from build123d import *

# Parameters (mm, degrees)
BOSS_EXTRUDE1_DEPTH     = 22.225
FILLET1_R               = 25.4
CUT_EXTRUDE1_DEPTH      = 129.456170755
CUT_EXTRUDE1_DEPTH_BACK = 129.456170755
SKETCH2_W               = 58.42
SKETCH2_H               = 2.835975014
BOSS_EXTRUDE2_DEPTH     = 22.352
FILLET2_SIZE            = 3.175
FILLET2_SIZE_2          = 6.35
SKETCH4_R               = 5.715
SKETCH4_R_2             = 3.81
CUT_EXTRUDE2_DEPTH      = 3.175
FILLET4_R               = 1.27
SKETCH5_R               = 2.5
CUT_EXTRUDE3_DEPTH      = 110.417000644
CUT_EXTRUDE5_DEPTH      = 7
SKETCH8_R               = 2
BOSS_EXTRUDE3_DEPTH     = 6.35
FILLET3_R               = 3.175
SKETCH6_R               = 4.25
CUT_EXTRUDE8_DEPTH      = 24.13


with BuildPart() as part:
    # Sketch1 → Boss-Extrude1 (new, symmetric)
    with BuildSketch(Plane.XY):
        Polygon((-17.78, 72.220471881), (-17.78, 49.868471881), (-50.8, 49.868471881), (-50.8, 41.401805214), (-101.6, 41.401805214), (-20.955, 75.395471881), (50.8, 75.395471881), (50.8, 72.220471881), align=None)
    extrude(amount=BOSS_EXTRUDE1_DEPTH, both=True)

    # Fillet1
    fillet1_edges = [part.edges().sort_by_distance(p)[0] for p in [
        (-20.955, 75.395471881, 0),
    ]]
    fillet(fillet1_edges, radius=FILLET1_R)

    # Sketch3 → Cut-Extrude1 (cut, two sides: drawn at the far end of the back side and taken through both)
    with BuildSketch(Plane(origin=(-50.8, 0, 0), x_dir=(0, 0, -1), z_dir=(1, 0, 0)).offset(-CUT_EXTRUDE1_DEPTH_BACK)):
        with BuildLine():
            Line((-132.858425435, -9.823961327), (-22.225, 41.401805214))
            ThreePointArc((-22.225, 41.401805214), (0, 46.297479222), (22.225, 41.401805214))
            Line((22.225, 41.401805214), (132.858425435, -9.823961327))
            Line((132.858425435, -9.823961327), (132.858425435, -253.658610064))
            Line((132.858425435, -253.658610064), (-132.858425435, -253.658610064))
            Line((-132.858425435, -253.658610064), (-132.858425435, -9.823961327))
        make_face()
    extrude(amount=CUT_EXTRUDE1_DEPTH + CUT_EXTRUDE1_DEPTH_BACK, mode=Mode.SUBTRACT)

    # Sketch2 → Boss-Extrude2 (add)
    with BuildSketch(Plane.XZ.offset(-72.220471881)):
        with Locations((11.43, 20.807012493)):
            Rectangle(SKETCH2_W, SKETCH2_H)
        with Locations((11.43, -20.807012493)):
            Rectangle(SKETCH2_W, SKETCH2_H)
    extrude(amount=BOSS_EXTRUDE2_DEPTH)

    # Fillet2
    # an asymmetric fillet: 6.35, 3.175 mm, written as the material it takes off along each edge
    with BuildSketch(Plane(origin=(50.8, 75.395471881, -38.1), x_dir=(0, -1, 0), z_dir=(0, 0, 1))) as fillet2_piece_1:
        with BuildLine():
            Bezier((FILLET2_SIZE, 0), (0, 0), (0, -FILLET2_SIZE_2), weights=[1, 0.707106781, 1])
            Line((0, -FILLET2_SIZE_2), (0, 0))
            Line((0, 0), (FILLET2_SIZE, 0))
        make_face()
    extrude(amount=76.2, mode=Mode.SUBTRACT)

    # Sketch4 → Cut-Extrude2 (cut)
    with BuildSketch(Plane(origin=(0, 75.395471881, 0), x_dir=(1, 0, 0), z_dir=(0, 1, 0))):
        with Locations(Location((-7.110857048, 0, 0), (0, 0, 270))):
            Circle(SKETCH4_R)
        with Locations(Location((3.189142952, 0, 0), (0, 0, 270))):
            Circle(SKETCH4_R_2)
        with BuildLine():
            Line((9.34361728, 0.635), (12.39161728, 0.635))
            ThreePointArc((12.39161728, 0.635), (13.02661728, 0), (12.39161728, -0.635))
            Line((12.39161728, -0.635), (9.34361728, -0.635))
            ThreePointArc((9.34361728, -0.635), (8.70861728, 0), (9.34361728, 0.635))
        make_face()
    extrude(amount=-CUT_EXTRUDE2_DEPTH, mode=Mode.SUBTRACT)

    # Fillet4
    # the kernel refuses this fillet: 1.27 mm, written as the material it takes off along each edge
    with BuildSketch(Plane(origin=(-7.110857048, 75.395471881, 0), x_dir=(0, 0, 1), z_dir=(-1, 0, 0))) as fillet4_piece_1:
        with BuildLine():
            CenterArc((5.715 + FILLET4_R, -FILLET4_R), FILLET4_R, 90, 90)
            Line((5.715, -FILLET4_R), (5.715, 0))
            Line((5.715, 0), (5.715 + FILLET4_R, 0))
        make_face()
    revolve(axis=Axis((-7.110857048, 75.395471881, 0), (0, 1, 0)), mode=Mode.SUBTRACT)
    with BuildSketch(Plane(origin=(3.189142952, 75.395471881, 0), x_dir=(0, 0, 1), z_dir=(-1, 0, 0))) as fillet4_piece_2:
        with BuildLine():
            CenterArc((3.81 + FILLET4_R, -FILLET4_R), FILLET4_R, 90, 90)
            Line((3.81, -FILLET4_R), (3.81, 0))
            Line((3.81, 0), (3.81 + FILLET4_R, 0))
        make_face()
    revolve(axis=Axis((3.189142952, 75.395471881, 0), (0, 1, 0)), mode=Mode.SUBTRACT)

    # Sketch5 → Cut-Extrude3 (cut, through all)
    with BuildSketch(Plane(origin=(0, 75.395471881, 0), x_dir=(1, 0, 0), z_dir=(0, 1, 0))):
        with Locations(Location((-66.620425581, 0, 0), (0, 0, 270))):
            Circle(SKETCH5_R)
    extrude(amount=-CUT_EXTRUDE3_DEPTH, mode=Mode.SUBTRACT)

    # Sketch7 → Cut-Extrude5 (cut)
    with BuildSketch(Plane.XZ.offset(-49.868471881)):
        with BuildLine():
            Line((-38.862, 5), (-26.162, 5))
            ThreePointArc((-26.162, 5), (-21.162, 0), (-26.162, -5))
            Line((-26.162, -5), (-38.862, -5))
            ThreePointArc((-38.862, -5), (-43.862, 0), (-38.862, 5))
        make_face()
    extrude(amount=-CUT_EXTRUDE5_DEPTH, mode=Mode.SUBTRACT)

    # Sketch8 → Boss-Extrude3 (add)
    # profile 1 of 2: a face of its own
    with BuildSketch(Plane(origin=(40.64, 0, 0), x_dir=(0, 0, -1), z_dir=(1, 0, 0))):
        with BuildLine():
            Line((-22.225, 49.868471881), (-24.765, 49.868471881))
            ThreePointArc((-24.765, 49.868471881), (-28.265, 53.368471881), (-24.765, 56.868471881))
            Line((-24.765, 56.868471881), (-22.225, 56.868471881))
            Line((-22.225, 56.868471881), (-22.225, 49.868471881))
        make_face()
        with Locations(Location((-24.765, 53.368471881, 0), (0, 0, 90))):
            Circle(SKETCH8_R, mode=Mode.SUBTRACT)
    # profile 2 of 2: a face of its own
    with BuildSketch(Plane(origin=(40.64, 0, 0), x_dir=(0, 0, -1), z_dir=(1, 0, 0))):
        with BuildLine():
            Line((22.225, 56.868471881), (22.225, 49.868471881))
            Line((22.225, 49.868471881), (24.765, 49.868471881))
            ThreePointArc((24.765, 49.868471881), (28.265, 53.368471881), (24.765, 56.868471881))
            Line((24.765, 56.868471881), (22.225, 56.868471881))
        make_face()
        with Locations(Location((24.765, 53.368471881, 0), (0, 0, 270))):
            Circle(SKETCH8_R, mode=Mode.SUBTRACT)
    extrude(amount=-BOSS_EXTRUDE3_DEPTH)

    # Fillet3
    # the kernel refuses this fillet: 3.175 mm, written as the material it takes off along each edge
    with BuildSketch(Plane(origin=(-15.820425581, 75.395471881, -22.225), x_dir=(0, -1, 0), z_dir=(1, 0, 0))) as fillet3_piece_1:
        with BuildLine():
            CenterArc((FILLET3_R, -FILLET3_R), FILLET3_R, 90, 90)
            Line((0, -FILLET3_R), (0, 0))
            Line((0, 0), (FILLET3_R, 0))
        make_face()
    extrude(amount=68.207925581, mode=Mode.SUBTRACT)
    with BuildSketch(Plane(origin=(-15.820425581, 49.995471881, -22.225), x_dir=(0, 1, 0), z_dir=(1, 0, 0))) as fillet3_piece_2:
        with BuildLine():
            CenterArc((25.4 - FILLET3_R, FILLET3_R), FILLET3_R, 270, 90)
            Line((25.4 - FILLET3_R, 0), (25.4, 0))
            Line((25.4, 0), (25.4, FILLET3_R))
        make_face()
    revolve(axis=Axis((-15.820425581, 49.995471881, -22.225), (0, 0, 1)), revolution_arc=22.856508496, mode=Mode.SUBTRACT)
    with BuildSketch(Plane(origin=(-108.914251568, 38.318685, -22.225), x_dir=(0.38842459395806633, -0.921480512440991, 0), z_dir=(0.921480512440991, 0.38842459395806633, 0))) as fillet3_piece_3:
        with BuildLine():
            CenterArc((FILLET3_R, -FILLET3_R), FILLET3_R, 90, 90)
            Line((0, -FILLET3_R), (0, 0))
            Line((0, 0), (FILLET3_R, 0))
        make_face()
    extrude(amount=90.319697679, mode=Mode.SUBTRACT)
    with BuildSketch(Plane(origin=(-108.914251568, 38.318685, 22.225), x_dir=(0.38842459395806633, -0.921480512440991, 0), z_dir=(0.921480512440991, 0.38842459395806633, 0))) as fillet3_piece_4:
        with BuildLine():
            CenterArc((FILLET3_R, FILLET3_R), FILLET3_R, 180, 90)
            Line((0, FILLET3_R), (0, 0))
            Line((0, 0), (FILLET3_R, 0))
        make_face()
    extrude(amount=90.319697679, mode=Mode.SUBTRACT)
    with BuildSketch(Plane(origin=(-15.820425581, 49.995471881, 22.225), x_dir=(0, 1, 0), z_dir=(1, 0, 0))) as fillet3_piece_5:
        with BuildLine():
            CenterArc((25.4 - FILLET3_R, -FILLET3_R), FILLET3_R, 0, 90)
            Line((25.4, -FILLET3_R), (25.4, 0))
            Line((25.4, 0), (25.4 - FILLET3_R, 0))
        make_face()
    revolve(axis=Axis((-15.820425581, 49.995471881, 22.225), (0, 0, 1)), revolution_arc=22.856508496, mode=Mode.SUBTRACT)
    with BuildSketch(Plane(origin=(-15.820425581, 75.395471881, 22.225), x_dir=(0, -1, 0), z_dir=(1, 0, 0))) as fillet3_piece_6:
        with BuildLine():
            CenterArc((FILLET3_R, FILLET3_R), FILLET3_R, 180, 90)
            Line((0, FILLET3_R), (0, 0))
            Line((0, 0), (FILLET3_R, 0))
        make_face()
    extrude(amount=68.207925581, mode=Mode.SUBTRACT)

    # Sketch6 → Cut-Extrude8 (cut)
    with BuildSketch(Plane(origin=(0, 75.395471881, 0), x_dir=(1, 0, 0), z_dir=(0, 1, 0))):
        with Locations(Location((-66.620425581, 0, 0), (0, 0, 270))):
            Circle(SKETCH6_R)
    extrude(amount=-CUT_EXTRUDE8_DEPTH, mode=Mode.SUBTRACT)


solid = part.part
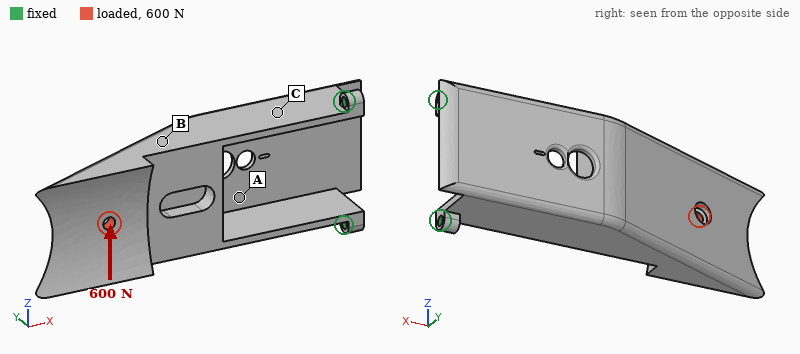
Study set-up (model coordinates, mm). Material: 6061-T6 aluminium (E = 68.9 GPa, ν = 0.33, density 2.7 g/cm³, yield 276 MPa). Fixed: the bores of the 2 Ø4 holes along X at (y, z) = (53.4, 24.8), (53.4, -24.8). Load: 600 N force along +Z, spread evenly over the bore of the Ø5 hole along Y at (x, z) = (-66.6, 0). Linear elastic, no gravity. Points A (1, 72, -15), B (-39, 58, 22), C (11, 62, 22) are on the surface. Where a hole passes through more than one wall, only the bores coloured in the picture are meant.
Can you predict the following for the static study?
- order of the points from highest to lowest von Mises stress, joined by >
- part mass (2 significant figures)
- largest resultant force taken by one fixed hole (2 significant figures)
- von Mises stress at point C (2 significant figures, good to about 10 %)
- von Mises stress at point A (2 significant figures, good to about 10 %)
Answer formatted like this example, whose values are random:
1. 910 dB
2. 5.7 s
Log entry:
1. C > A > B
2. 160 g
3. 1.4 kN
4. 55 MPa
5. 30 MPa
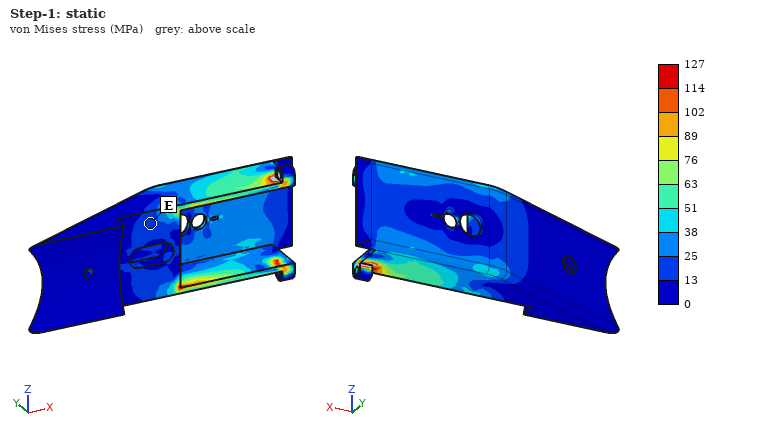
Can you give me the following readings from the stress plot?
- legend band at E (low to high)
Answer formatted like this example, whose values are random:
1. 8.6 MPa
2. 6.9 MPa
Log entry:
1. 13 to 25 MPa
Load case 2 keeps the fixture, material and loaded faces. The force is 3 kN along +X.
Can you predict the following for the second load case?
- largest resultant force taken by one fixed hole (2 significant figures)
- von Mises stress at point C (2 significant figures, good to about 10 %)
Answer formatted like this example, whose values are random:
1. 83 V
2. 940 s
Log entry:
1. 1.5 kN
2. 31 MPa
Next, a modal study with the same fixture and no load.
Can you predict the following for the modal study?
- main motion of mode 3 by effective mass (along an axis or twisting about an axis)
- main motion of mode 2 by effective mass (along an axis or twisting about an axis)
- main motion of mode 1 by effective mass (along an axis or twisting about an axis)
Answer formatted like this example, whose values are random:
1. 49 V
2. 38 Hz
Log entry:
1. along Z
2. along Z
3. along Y
